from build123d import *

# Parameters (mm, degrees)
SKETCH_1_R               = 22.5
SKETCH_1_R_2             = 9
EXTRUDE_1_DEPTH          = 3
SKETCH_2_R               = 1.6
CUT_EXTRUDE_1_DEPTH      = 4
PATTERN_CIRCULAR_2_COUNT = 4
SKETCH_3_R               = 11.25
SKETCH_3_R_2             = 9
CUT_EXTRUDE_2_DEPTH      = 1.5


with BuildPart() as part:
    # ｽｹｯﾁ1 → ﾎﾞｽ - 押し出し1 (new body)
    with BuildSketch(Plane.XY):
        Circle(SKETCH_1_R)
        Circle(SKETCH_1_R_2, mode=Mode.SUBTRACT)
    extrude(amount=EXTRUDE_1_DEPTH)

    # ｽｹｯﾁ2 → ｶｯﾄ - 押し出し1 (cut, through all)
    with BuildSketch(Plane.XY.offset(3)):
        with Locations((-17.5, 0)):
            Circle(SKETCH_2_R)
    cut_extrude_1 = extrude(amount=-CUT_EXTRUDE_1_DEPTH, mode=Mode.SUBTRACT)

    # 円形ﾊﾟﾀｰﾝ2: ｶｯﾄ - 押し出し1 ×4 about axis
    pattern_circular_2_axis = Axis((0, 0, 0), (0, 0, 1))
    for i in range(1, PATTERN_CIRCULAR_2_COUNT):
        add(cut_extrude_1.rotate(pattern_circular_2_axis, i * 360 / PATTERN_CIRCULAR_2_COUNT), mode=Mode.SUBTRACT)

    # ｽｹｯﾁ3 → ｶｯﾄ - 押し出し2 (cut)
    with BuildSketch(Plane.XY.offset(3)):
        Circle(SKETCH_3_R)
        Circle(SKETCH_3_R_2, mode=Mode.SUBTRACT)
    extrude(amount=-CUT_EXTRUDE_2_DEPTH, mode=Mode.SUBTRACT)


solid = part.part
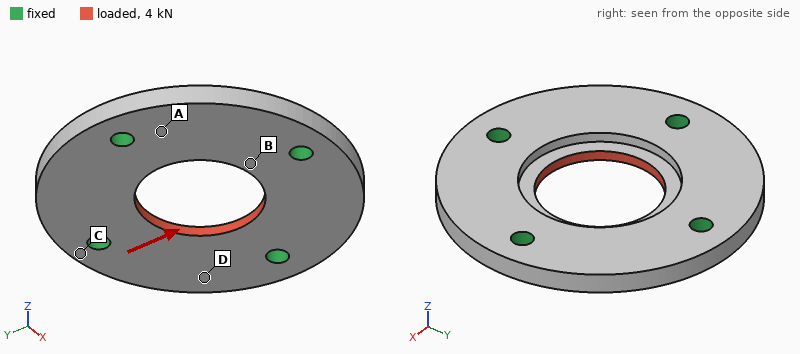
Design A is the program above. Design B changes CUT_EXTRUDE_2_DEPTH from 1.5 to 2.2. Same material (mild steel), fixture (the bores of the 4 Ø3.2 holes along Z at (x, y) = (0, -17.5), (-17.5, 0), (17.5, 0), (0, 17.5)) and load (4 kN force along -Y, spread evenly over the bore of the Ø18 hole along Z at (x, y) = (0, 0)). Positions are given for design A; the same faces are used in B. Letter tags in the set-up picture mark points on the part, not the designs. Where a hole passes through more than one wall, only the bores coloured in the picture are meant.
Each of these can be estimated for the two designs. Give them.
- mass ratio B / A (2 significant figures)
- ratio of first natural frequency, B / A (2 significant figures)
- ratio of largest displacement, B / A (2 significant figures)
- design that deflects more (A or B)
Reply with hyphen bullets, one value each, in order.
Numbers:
- 0.97
- 1.0
- 1.5
- B
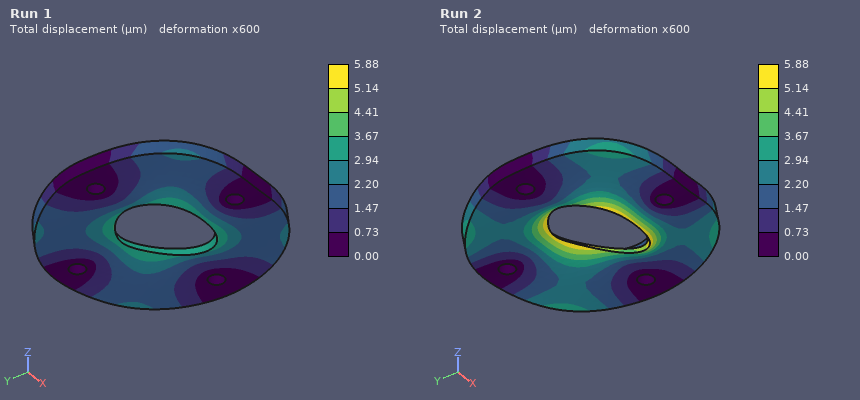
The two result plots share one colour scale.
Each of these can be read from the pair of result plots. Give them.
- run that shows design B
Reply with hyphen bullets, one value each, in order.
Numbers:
- Run 2
